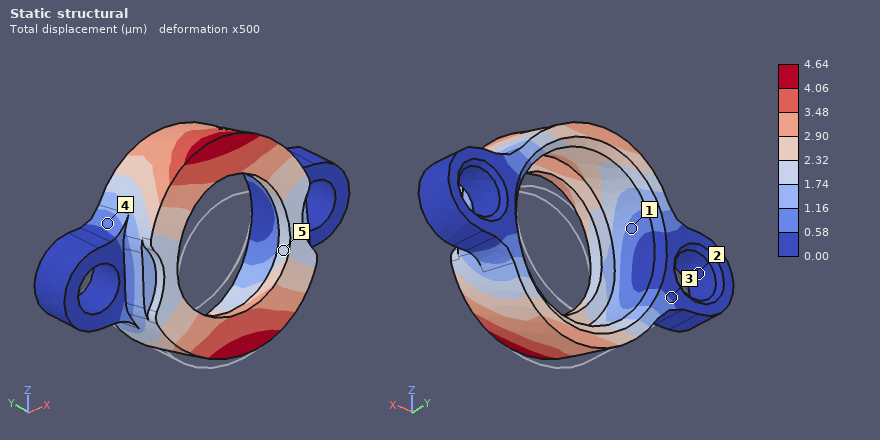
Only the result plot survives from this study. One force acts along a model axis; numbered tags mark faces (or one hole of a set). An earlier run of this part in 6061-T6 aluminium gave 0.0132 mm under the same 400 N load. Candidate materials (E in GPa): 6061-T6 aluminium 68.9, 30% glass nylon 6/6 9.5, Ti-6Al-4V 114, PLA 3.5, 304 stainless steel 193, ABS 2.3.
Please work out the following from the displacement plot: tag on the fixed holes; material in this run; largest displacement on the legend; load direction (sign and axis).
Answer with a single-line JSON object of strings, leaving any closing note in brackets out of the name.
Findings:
{"tag on the fixed holes": "2", "material in this run": "304 stainless steel", "largest displacement on the legend": "4.64 µm", "load direction": "+Z"}
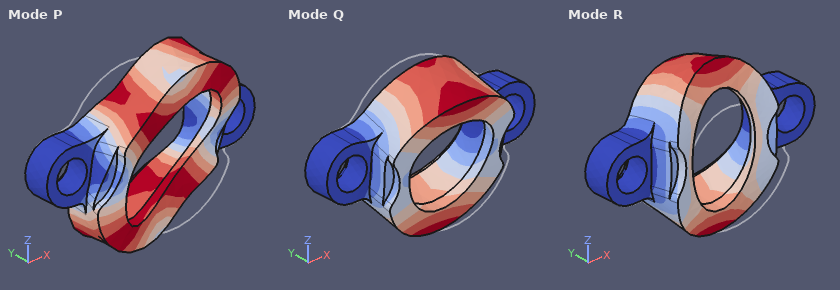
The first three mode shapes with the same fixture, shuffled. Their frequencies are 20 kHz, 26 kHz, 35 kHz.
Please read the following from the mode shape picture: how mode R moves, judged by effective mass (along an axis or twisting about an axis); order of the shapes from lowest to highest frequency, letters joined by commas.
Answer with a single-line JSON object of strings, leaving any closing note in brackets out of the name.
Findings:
{"how mode R moves, judged by effective mass": "along Y", "order of the shapes from lowest to highest frequency, letters joined by commas": "Q, R, P"}
